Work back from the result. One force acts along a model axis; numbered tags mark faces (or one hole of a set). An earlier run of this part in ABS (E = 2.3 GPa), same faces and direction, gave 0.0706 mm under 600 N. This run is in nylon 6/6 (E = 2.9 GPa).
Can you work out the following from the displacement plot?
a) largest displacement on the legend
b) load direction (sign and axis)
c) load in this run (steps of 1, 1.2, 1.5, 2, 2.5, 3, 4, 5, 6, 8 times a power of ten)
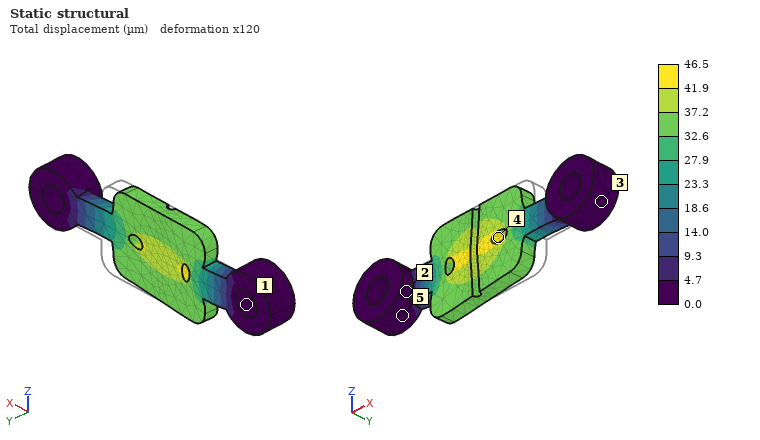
46.5 µm
-X
500 N
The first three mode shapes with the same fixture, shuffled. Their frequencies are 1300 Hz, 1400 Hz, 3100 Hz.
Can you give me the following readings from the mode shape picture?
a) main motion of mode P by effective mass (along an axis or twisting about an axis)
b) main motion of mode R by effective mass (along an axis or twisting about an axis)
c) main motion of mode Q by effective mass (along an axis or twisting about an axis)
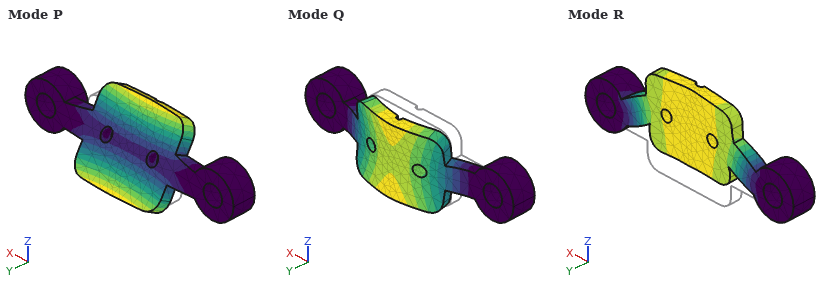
twisting about X
along Z
along Y
